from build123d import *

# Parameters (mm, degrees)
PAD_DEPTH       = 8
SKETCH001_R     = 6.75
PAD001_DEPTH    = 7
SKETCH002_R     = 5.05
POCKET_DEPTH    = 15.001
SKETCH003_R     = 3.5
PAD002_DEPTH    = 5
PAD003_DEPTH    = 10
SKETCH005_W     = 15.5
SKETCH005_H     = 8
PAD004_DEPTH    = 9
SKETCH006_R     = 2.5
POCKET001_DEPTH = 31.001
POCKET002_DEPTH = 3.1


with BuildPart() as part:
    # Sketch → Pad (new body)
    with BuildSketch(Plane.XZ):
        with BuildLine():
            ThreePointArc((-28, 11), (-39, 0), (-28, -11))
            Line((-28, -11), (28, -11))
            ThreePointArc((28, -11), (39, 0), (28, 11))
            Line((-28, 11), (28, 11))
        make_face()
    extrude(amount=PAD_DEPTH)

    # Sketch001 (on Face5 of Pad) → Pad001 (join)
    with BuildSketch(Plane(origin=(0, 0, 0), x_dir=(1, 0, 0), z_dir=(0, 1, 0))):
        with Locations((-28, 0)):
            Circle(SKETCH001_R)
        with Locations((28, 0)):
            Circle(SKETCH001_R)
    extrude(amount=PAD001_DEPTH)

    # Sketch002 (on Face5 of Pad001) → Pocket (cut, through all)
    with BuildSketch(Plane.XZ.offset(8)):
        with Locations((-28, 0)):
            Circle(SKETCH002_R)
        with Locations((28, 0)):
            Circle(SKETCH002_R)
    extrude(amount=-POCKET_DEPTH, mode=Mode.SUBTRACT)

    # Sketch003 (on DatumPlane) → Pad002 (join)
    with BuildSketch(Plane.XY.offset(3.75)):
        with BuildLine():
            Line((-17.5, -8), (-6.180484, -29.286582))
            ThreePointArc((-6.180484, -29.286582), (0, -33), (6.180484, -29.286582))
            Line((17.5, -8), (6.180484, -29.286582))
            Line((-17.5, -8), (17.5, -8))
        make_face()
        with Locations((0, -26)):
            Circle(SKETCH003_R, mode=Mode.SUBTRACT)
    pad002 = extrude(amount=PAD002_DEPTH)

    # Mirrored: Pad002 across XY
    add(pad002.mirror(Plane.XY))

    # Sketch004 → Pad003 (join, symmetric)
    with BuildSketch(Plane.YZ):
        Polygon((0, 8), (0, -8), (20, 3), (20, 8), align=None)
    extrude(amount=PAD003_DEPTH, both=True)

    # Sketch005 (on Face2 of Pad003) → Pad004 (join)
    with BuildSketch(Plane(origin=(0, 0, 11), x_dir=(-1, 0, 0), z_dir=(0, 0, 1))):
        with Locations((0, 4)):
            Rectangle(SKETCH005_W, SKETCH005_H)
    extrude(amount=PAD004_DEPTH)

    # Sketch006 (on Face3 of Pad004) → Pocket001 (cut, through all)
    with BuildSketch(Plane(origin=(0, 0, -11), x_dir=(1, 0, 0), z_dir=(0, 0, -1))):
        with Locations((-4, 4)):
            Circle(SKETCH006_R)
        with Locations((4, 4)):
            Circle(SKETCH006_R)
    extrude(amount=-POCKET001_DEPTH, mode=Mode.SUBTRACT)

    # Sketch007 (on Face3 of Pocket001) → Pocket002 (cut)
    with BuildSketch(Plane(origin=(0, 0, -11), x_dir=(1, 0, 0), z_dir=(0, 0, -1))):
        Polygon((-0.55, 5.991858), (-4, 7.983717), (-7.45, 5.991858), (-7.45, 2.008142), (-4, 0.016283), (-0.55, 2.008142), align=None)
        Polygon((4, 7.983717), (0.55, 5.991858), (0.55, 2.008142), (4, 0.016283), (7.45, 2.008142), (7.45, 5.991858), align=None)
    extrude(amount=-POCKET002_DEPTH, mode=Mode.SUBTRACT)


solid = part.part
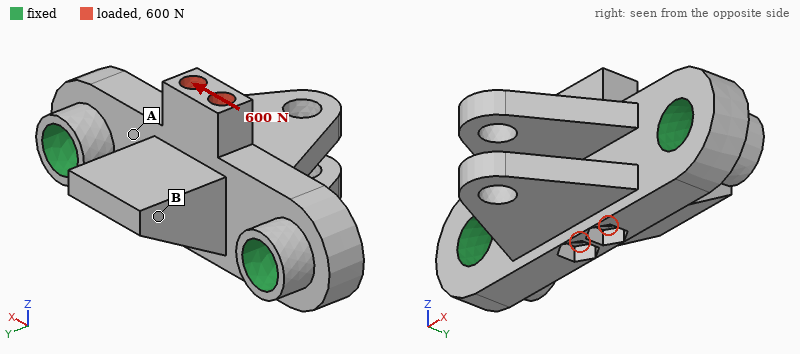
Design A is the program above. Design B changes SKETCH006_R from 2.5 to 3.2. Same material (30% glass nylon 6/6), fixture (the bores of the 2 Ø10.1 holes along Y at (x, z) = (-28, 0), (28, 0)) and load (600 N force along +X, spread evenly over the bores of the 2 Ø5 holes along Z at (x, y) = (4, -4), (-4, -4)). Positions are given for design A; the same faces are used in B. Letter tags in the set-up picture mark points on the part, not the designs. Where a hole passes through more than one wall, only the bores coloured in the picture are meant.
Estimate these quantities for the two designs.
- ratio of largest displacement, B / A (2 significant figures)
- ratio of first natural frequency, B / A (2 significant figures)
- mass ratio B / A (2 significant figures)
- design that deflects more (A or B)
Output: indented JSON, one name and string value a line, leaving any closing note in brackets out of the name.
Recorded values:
{
  "ratio of largest displacement, B / A": "1.4",
  "ratio of first natural frequency, B / A": "0.99",
  "mass ratio B / A": "0.97",
  "design that deflects more": "B"
}
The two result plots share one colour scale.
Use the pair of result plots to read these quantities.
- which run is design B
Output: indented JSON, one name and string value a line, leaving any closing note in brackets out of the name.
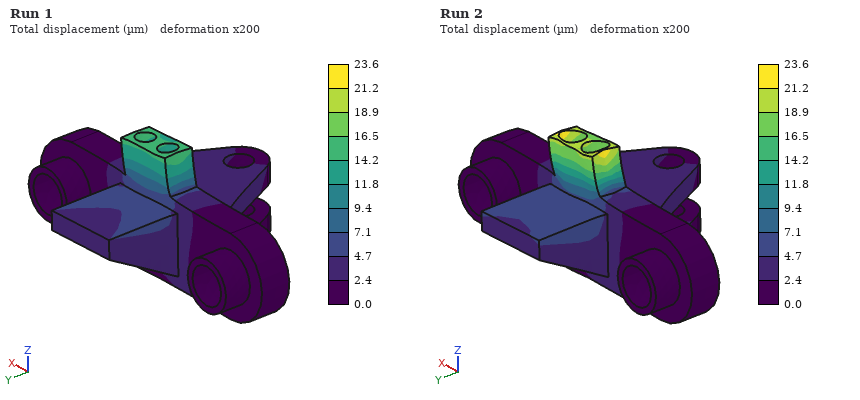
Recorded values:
{
  "which run is design B": "Run 2"
}
